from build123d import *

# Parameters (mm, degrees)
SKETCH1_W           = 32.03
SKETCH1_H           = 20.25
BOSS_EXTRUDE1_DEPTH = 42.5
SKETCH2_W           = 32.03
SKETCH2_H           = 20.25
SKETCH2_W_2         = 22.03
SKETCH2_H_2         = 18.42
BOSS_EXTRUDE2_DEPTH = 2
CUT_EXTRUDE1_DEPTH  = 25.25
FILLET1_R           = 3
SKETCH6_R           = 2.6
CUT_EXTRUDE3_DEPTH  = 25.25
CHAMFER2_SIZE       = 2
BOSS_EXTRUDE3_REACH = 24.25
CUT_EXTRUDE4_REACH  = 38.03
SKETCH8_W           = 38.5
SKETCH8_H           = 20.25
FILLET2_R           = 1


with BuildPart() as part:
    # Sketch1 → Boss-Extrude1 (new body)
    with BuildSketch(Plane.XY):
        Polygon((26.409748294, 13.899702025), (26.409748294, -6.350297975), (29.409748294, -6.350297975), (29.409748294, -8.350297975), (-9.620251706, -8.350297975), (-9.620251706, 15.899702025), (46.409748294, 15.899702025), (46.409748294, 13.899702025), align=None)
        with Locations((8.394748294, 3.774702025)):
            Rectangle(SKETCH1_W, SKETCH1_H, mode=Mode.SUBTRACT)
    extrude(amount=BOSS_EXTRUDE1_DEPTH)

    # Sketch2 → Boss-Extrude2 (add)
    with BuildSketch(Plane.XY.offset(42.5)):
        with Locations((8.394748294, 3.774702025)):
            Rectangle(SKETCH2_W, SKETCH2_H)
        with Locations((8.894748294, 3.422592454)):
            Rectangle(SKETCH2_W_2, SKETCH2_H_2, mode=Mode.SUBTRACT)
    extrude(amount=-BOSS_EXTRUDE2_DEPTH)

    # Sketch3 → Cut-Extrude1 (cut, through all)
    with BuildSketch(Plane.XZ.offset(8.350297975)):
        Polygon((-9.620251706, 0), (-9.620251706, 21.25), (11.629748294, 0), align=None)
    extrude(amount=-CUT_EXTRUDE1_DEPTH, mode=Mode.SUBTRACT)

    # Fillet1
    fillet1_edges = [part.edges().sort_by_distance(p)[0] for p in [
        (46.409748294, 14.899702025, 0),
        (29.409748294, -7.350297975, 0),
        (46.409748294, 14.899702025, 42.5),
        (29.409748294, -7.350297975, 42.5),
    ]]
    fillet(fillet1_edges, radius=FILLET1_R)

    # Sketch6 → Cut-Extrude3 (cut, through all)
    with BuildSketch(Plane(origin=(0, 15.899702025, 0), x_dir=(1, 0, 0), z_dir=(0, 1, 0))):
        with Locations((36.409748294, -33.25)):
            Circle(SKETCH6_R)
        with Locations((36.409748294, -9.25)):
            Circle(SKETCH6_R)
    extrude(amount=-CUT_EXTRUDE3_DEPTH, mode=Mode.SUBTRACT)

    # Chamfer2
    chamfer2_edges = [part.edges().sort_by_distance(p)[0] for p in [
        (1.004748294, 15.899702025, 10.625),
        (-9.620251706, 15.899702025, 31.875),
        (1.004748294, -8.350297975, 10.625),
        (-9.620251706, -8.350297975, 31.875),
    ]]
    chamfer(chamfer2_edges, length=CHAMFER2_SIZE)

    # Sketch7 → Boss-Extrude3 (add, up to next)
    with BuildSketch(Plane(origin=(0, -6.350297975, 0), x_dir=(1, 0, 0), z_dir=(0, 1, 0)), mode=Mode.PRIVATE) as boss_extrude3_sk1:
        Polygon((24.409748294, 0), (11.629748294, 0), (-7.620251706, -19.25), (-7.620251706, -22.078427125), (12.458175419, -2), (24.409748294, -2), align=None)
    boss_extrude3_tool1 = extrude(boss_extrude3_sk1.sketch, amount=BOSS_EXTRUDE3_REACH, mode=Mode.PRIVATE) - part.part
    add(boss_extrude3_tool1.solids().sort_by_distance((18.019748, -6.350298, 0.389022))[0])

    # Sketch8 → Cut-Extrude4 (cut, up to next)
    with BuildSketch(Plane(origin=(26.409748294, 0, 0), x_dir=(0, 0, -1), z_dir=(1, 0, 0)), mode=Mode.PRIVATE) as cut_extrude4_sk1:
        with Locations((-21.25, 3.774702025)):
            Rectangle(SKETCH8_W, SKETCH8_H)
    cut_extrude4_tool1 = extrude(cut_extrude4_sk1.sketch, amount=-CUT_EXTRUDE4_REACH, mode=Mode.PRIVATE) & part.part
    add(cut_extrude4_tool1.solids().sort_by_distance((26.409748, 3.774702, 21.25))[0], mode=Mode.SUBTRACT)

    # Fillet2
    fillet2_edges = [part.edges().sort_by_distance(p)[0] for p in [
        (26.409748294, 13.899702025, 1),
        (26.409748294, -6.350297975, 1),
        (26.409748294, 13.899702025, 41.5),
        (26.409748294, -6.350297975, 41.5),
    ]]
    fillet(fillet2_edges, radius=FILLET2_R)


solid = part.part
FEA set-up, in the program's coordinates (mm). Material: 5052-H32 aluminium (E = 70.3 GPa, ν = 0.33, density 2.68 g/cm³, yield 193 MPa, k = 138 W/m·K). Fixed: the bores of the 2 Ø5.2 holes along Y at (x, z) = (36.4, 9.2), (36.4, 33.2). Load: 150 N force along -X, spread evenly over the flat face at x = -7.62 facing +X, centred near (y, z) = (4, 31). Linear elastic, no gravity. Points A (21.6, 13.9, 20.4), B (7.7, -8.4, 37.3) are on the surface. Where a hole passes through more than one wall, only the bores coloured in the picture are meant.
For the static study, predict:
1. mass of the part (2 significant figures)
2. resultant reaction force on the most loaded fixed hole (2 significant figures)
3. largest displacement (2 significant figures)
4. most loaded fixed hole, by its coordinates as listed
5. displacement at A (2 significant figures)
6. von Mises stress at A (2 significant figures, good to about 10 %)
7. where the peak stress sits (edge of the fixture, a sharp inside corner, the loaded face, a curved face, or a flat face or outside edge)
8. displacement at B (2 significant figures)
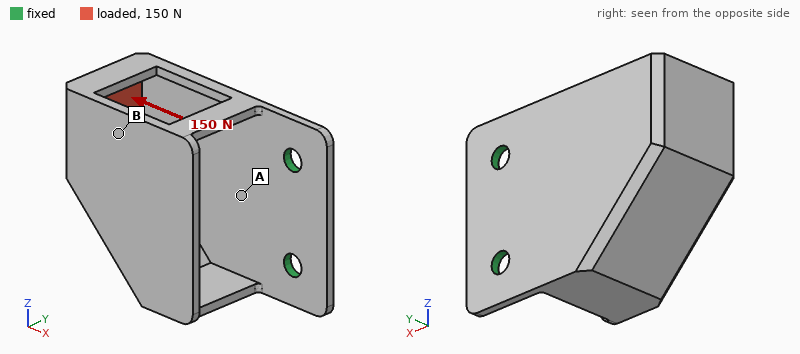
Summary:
27 g
130 N
0.48 mm
(36.4, 33.2)
0.073 mm
27 MPa
a curved face
0.35 mm
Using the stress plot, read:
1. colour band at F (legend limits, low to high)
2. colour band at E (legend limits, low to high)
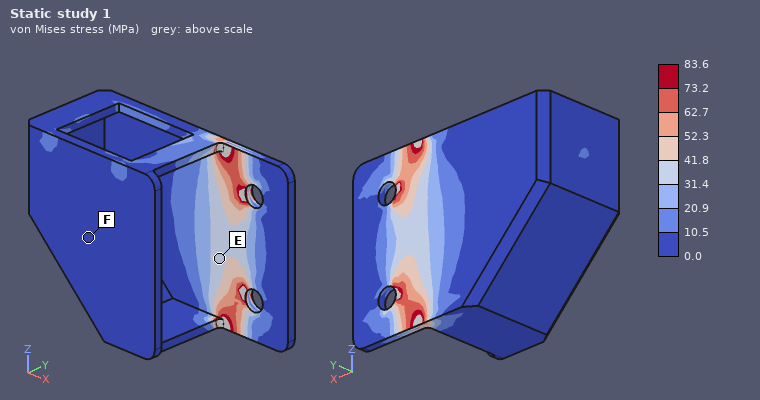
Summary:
0.0 to 10.5 MPa
31.4 to 41.8 MPa
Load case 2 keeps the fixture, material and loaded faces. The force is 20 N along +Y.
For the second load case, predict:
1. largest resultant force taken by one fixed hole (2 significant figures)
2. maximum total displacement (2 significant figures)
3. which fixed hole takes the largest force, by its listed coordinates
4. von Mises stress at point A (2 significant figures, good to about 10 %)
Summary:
16 N
0.21 mm
(36.4, 33.2)
11 MPa
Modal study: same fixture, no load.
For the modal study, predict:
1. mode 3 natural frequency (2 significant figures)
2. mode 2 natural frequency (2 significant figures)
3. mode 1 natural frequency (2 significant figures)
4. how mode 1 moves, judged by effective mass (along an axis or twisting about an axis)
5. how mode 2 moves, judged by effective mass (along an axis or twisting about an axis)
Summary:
3000 Hz
1200 Hz
480 Hz
along Y
along Z
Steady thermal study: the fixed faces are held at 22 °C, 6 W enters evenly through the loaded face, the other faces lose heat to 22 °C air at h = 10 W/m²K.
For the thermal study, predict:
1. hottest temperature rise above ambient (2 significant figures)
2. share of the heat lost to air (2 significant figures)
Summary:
19 K
18 %
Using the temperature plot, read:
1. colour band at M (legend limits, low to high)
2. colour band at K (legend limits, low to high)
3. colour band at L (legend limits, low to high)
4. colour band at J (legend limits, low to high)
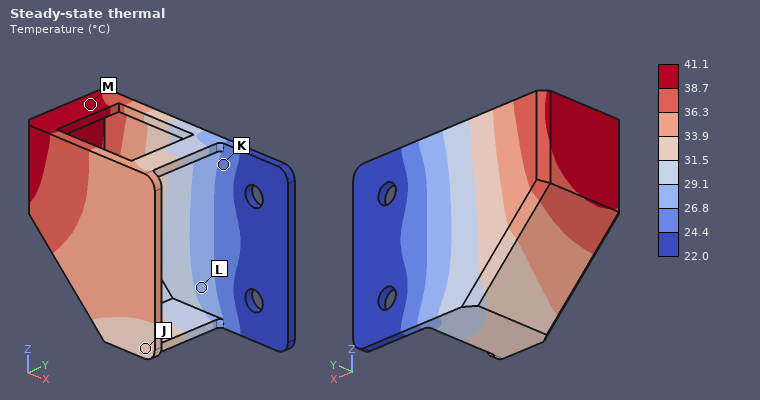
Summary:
38.7 to 41.1 °C
24.4 to 26.8 °C
26.8 to 29.1 °C
31.5 to 33.9 °C
